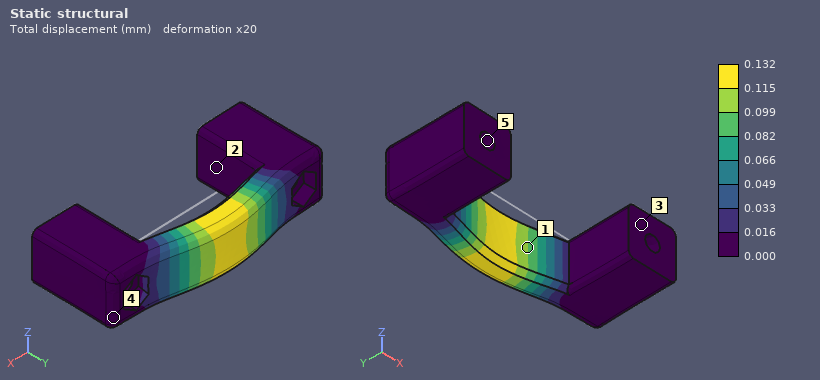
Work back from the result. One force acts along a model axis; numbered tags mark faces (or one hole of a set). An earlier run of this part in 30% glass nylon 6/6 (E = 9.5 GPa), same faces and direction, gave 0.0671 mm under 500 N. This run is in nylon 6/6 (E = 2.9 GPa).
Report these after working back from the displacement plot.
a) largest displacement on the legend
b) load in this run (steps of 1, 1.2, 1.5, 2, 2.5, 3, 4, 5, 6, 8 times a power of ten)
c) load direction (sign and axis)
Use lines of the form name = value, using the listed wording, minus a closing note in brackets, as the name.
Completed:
largest displacement on the legend = 0.132 mm
load in this run = 300 N
load direction = +Y
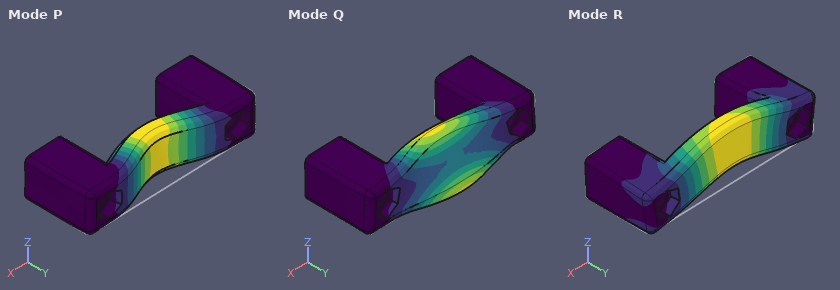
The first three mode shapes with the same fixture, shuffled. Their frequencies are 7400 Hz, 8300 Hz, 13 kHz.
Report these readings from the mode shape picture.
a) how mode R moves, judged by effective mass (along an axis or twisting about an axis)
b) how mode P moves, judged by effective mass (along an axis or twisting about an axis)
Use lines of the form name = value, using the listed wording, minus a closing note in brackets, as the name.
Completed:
how mode R moves, judged by effective mass = along Z
how mode P moves, judged by effective mass = along Y
